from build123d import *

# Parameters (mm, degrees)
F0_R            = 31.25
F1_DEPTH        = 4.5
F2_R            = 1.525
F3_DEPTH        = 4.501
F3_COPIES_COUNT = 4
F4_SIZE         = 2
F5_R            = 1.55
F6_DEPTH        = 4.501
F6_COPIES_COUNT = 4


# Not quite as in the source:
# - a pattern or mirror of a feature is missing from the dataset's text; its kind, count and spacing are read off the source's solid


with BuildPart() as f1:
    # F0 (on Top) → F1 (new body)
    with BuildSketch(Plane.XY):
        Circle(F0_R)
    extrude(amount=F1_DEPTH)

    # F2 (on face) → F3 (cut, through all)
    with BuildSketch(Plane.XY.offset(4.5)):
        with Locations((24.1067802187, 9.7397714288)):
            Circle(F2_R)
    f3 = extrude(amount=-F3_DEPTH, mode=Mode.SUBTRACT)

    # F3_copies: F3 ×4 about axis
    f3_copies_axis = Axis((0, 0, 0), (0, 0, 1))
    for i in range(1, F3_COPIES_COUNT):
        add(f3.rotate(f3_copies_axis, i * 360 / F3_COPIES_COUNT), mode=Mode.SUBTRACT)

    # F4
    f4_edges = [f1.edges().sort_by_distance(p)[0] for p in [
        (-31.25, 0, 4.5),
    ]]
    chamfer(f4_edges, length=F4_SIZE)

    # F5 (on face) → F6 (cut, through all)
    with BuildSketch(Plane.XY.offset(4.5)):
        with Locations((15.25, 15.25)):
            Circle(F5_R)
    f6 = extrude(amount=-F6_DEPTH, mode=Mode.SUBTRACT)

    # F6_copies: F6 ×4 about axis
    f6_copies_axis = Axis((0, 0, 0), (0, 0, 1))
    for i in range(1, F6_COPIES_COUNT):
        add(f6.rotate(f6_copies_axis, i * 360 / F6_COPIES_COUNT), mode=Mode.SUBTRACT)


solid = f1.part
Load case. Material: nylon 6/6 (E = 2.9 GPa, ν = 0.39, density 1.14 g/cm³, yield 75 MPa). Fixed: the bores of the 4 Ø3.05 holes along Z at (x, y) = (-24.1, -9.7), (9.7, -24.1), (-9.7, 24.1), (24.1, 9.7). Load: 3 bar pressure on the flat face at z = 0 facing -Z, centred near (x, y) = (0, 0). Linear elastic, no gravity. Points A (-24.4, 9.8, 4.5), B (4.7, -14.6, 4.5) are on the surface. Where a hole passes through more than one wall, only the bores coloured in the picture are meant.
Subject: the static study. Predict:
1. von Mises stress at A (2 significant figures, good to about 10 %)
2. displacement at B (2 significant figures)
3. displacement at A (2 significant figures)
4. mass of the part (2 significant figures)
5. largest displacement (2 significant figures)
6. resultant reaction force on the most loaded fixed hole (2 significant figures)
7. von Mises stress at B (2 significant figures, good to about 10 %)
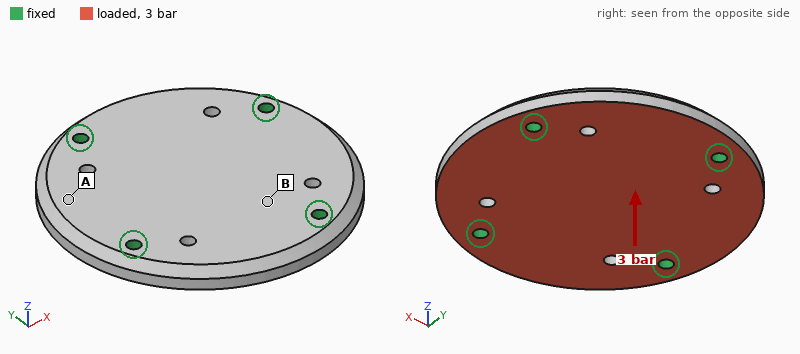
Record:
6.1 MPa
0.096 mm
0.11 mm
15 g
0.16 mm
230 N
2.7 MPa
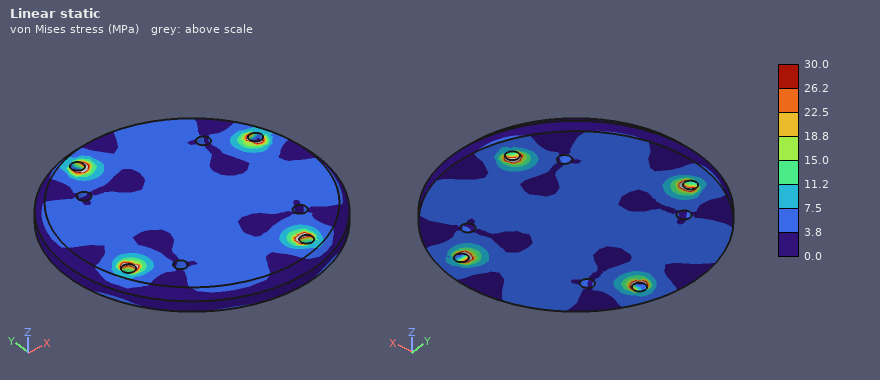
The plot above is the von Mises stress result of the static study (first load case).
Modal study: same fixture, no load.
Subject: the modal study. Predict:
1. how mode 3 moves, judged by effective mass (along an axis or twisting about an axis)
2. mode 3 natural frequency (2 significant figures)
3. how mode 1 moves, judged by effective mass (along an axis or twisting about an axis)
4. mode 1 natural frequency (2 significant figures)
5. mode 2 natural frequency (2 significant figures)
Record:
twisting about X
4100 Hz
along Z
3600 Hz
3800 Hz
